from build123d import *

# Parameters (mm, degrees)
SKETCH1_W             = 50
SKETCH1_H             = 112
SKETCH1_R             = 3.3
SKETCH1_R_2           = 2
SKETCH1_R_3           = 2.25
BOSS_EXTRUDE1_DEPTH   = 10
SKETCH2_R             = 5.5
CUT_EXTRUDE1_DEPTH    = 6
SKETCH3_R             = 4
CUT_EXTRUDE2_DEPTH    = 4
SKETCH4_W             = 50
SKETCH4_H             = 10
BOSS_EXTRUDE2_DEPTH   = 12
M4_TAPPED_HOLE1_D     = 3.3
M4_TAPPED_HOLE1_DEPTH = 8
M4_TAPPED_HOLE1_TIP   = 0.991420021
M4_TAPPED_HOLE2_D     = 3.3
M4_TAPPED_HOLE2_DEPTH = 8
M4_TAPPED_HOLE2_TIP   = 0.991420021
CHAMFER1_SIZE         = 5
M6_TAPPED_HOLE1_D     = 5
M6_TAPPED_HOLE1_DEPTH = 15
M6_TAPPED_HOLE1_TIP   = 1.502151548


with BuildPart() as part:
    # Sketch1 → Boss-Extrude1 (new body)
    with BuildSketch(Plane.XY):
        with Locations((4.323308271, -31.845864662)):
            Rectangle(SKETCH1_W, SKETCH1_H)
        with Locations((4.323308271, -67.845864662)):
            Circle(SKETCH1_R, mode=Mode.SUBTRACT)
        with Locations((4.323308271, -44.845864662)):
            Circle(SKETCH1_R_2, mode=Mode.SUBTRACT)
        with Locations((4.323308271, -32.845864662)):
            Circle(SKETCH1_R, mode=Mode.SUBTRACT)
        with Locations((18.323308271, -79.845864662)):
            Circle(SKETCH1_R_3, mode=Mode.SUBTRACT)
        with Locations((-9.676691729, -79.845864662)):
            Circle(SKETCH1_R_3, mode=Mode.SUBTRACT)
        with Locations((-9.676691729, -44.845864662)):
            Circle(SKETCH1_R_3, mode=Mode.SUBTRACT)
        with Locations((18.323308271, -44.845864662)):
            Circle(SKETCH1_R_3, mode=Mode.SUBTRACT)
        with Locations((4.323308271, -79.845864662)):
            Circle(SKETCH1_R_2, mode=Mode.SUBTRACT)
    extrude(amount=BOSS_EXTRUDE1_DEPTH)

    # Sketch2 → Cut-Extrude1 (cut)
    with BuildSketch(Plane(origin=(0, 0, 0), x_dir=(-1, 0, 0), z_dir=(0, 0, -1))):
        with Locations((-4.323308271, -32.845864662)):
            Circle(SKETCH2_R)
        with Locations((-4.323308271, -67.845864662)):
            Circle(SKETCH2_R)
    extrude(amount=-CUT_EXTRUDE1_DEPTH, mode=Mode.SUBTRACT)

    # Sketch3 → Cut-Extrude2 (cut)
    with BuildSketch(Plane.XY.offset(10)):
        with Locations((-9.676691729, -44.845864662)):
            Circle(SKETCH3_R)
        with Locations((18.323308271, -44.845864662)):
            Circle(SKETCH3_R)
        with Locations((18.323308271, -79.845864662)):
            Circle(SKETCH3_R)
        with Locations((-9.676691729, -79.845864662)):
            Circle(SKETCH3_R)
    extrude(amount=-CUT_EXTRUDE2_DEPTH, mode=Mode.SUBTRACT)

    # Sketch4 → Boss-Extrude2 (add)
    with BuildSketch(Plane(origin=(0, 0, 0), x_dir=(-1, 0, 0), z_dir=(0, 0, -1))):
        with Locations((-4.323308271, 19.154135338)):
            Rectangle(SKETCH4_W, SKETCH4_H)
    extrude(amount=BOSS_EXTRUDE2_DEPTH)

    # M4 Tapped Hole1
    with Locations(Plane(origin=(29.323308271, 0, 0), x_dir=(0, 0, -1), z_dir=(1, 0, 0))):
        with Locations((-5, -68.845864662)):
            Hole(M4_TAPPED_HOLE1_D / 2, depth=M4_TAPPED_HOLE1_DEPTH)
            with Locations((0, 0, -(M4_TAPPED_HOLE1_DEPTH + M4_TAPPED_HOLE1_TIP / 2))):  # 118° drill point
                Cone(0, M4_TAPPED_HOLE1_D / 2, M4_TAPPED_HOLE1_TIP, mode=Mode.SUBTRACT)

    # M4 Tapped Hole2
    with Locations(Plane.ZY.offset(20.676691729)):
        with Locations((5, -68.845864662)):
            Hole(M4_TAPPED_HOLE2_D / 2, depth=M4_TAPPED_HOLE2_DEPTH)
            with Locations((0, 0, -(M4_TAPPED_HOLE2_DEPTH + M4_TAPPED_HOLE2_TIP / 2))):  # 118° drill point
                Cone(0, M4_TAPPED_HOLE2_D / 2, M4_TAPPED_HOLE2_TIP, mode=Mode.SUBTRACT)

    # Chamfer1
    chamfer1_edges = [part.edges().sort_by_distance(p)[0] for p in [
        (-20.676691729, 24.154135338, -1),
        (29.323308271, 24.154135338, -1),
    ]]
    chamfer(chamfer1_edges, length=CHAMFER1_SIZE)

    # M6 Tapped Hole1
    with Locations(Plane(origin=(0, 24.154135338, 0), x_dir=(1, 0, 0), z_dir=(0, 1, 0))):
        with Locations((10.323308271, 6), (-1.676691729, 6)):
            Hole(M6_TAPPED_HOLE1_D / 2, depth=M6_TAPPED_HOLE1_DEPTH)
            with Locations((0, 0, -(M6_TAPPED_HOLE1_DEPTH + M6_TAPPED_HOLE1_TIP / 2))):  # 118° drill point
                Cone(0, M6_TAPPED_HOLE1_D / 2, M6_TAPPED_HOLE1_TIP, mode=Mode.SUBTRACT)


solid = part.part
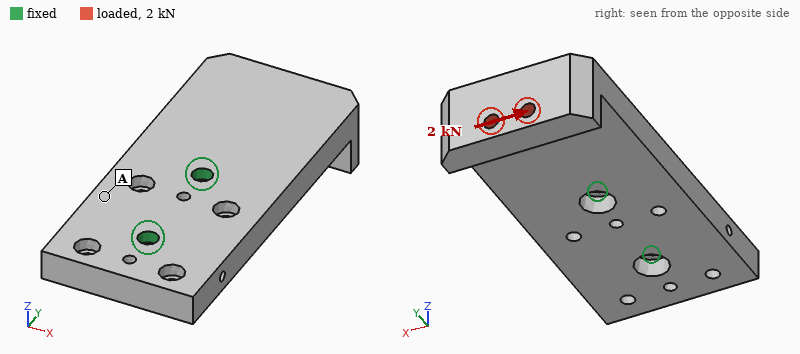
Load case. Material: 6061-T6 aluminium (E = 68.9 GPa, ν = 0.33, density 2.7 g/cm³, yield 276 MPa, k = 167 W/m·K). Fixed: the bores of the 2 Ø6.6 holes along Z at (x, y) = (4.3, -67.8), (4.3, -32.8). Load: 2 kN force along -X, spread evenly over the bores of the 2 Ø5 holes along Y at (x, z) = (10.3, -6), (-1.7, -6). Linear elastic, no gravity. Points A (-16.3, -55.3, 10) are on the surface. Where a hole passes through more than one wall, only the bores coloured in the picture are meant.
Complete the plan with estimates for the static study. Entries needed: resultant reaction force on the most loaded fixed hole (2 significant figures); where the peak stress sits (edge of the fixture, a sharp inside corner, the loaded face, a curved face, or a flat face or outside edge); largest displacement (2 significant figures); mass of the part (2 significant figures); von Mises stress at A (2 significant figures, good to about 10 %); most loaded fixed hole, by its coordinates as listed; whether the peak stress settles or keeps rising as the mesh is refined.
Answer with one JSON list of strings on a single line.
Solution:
["4.5 kN", "edge of the fixture", "0.21 mm", "160 g", "25 MPa", "(4.3, -32.8)", "keeps rising"]
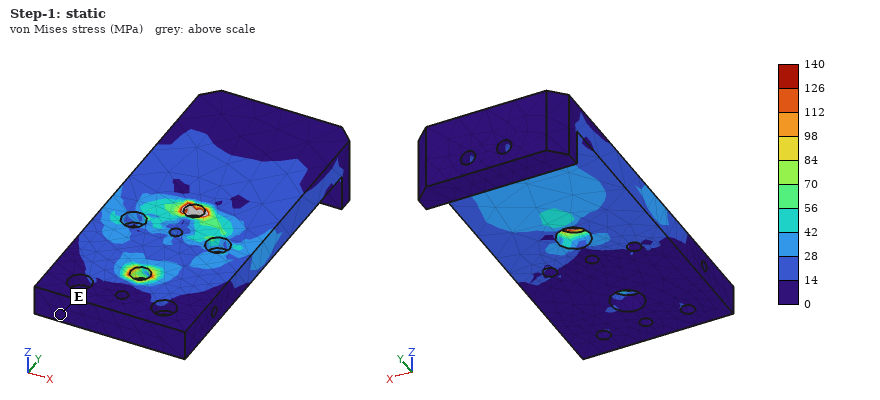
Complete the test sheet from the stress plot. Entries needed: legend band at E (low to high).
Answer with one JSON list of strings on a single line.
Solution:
["0 to 14 MPa"]
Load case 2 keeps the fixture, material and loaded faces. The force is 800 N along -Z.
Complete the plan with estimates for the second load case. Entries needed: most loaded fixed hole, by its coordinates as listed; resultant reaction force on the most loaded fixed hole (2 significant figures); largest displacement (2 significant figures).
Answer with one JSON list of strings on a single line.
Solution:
["(4.3, -32.8)", "2.3 kN", "0.25 mm"]
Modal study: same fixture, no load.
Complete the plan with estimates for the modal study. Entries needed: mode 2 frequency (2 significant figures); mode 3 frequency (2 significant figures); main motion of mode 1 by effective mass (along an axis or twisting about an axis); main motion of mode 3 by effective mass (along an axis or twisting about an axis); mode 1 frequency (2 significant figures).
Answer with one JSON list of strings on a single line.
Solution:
["2500 Hz", "4400 Hz", "along Z", "along X", "1500 Hz"]
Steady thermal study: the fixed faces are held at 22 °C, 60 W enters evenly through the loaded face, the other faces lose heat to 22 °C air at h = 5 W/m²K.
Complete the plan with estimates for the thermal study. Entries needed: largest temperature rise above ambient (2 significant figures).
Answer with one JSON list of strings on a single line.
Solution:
["58 K"]
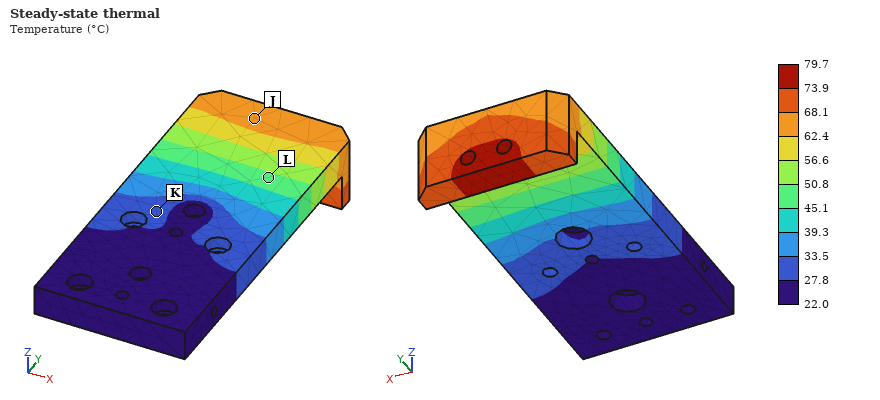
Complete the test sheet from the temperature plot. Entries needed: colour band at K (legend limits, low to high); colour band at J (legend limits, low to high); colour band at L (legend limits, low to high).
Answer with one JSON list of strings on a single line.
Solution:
["27.8 to 33.5 °C", "62.4 to 68.1 °C", "45.1 to 50.8 °C"]
